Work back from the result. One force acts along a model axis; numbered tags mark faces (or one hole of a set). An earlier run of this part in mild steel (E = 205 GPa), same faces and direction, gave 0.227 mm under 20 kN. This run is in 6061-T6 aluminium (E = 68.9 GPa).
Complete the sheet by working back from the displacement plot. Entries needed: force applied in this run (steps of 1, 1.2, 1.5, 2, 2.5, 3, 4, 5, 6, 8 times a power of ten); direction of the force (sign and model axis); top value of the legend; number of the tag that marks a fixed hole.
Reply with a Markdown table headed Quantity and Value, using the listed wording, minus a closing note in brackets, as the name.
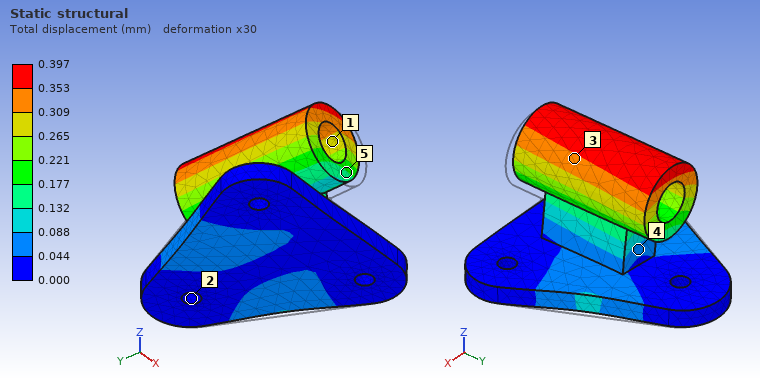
| Quantity | Value |
|---|---|
| force applied in this run | 12 kN |
| direction of the force | -X |
| top value of the legend | 0.397 mm |
| number of the tag that marks a fixed hole | 2 |
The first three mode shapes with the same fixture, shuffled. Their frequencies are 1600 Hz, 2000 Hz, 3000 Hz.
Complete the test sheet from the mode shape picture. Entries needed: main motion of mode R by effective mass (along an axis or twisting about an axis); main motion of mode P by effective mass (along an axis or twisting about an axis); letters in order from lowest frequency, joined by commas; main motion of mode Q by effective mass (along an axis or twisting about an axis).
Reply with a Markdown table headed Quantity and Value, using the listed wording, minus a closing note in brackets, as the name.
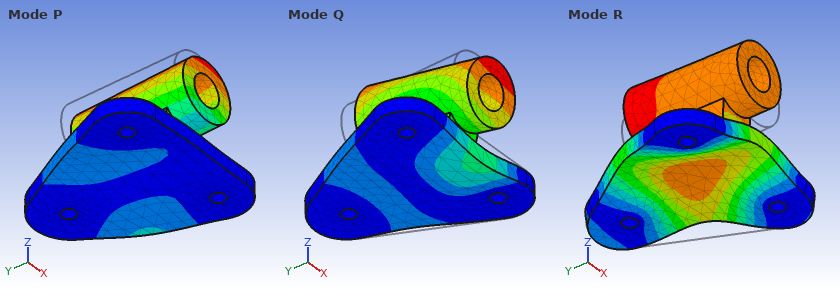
| Quantity | Value |
|---|---|
| main motion of mode R by effective mass | along Z |
| main motion of mode P by effective mass | along X |
| letters in order from lowest frequency, joined by commas | P, Q, R |
| main motion of mode Q by effective mass | along Y |
